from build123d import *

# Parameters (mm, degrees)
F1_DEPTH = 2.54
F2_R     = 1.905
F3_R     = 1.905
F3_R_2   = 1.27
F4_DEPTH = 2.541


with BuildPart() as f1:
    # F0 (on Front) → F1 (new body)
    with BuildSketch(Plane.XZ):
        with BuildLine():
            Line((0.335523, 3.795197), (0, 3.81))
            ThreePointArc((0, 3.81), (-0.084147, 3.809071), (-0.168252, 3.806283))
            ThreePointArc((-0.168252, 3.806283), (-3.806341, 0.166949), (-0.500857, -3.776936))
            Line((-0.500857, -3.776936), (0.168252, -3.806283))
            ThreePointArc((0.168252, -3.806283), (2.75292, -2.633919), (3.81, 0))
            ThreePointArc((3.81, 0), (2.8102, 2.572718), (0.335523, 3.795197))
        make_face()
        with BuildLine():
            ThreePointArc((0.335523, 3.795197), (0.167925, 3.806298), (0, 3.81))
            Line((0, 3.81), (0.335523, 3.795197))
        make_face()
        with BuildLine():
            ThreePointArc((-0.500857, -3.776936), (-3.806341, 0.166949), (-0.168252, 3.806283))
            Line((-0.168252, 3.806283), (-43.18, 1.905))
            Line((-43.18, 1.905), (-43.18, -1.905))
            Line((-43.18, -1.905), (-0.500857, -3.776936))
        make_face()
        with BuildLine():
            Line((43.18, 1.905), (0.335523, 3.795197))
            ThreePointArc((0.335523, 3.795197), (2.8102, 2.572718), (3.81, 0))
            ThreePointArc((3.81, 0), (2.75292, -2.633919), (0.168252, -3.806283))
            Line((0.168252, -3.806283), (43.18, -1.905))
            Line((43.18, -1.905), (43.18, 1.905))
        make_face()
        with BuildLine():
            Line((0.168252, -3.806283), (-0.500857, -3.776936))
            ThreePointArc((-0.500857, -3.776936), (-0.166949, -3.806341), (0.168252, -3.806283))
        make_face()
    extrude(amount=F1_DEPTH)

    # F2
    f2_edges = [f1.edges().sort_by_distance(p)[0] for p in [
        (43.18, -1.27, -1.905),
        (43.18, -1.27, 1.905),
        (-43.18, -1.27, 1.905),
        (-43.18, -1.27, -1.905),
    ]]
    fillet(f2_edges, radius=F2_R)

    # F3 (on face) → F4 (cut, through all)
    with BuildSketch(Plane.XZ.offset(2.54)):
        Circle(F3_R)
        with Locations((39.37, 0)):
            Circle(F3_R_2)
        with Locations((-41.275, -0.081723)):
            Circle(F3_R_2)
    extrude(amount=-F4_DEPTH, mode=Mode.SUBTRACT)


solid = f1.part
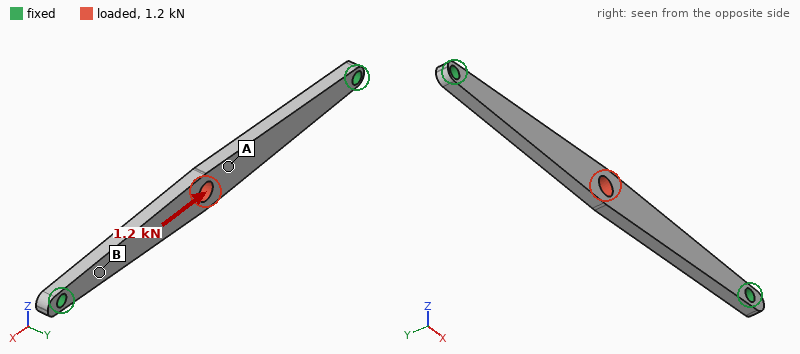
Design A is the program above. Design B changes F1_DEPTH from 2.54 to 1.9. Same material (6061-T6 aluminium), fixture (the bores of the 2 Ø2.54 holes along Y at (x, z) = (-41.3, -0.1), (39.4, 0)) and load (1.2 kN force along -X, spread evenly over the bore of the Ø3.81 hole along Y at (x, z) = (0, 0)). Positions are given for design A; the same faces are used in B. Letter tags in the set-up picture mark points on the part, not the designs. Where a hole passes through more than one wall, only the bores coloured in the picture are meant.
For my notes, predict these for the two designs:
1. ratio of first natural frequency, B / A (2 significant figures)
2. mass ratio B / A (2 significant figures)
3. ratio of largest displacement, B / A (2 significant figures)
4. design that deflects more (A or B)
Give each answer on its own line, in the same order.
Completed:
0.75
0.75
1.3
B
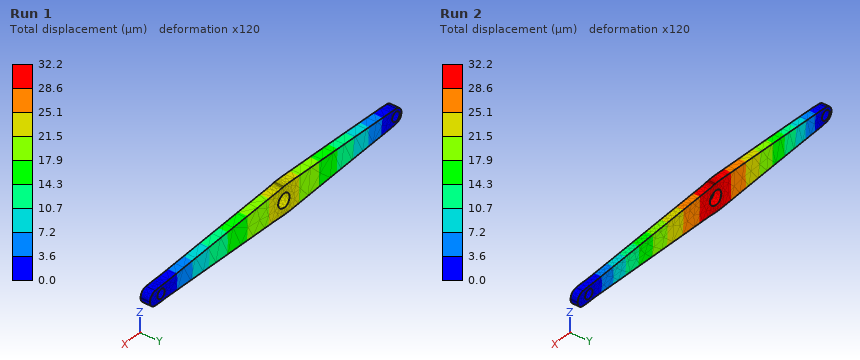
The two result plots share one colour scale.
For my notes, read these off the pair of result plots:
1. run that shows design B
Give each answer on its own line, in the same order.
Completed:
Run 2
